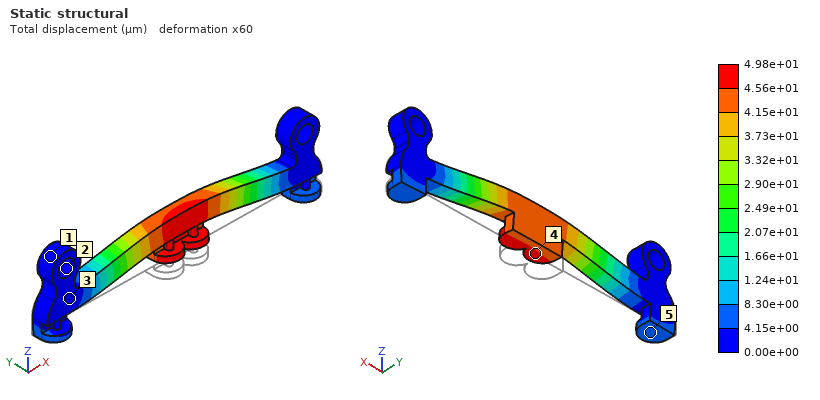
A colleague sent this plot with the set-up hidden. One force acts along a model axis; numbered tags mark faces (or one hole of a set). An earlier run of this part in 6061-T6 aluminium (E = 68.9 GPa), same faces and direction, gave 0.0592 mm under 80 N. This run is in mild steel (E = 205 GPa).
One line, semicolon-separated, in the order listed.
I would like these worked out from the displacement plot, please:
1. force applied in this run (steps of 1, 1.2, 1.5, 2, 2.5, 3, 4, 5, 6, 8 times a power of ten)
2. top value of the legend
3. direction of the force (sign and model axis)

200 N; 4.98e+01 µm; +Z
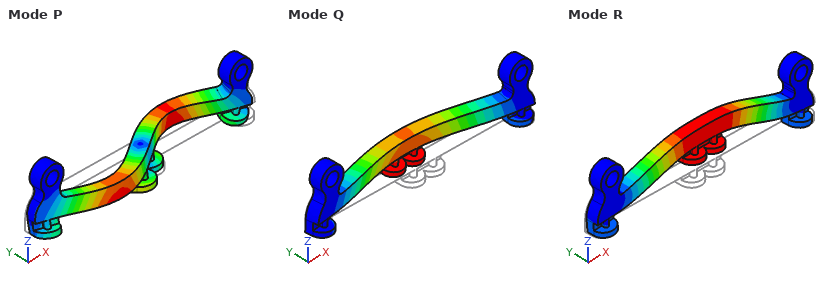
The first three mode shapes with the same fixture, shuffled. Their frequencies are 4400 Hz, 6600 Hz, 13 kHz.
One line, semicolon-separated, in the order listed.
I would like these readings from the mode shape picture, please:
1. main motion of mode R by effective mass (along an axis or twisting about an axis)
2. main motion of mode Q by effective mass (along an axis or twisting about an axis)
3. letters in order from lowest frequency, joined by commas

along Z; along Y; Q, R, P
